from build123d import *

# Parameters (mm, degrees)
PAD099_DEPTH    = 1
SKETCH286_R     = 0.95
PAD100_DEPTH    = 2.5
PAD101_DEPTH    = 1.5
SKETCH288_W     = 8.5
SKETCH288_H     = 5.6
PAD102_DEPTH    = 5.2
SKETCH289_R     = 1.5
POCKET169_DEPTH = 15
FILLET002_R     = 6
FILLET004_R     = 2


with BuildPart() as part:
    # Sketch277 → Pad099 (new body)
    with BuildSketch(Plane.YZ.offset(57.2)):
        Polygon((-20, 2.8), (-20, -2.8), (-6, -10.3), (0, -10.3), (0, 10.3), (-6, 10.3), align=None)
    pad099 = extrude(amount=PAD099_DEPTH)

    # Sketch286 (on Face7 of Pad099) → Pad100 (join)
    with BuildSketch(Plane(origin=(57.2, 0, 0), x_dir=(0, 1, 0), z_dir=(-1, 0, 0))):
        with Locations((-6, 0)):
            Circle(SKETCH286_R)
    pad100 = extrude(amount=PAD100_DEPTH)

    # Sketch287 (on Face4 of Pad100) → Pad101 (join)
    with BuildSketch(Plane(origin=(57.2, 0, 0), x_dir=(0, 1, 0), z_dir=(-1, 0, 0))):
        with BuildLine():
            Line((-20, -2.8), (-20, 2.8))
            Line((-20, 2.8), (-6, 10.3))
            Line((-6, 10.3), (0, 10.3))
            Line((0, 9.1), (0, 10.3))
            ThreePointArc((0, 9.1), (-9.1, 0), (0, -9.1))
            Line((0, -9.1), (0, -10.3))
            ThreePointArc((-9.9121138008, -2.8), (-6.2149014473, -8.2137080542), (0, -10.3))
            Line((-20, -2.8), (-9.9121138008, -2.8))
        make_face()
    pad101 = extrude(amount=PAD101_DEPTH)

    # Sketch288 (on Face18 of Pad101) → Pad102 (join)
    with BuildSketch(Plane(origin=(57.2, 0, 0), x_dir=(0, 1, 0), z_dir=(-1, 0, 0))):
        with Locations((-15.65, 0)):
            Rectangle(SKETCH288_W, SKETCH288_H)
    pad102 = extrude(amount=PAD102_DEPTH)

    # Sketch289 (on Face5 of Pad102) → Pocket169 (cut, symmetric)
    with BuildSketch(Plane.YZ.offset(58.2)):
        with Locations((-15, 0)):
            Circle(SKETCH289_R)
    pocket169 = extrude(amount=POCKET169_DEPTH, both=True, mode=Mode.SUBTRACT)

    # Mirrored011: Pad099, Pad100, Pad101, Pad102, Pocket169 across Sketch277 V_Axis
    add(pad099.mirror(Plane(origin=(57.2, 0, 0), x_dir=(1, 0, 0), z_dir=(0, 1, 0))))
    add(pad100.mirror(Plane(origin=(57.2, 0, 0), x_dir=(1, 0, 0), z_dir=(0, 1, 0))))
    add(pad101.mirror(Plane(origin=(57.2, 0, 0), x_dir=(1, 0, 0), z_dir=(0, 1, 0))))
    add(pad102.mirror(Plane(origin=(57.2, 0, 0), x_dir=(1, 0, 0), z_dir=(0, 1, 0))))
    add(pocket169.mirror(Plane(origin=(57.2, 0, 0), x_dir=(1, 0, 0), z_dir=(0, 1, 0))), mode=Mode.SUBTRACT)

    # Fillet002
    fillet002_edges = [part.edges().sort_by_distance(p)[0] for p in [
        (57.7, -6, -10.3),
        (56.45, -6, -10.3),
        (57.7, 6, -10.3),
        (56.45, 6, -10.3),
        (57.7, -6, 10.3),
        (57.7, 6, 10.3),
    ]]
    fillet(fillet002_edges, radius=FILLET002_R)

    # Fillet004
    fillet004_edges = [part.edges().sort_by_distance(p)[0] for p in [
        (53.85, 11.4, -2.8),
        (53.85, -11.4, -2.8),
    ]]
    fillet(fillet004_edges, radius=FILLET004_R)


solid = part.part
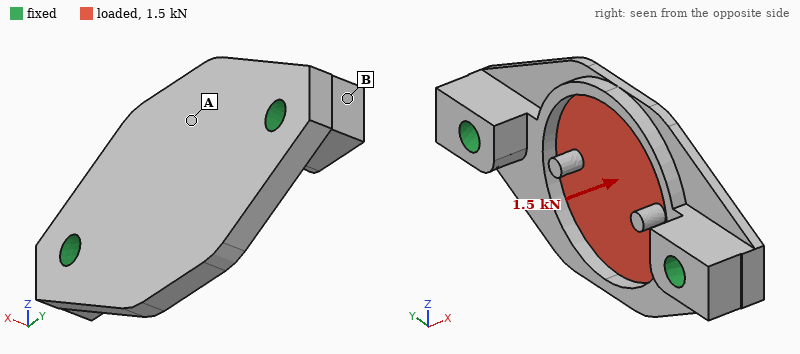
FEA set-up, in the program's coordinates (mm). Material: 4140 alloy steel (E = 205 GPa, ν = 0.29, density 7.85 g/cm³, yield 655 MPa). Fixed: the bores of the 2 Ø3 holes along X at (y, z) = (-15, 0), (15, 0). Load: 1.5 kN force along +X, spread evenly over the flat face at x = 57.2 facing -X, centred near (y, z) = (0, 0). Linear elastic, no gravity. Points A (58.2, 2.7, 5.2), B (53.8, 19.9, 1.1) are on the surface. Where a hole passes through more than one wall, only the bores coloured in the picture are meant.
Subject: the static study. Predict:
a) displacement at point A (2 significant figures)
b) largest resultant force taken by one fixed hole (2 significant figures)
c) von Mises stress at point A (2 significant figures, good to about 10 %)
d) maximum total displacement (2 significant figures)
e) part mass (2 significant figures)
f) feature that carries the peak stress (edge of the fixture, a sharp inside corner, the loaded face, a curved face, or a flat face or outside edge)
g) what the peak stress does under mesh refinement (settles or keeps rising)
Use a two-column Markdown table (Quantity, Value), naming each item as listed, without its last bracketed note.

| Quantity | Value |
|---|---|
| displacement at point A | 82 µm |
| largest resultant force taken by one fixed hole | 1.0 kN |
| von Mises stress at point A | 270 MPa |
| maximum total displacement | 97 µm |
| part mass | 10 g |
| feature that carries the peak stress | a sharp inside corner |
| what the peak stress does under mesh refinement | keeps rising |
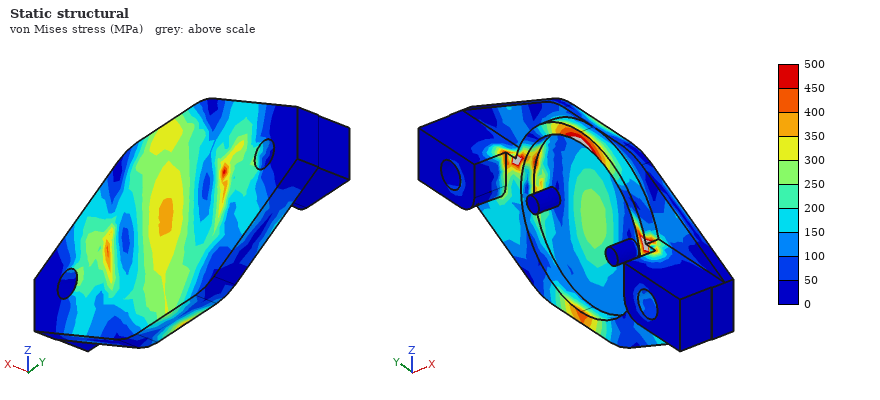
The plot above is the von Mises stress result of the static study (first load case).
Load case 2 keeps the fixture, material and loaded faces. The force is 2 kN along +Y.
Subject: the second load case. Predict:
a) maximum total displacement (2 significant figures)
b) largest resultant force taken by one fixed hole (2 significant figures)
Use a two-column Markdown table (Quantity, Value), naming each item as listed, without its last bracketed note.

| Quantity | Value |
|---|---|
| maximum total displacement | 4.4 µm |
| largest resultant force taken by one fixed hole | 1.0 kN |
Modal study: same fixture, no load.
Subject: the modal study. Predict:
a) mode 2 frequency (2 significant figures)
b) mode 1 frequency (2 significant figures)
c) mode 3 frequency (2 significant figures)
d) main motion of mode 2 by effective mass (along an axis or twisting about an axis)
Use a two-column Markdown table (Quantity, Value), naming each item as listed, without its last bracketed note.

| Quantity | Value |
|---|---|
| mode 2 frequency | 14 kHz |
| mode 1 frequency | 11 kHz |
| mode 3 frequency | 24 kHz |
| main motion of mode 2 by effective mass | along X |
